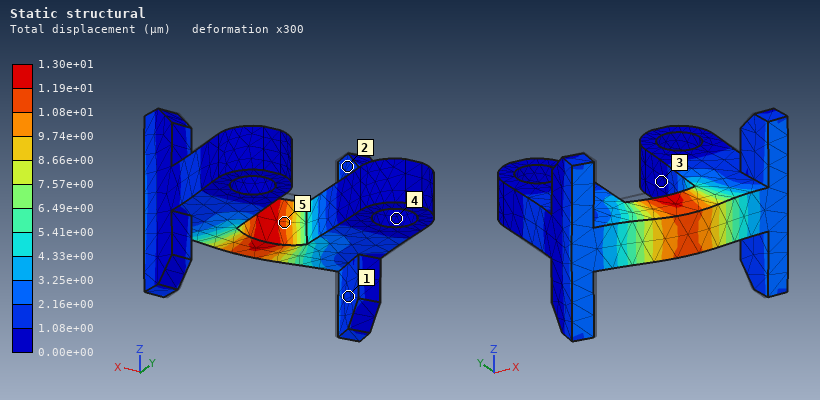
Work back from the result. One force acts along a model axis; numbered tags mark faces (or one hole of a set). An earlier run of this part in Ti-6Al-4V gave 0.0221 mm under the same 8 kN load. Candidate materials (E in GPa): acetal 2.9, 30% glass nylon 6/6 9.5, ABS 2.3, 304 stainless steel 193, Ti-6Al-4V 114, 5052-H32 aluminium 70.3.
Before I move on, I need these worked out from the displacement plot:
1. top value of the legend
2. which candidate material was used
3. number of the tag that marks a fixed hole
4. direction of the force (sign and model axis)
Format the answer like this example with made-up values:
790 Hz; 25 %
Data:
1.30e+01 µm; 304 stainless steel; 4; -Y
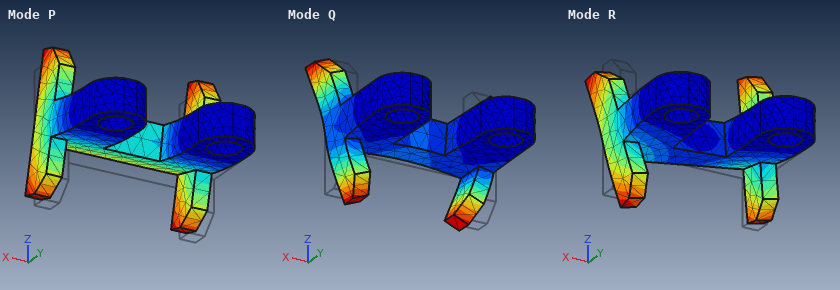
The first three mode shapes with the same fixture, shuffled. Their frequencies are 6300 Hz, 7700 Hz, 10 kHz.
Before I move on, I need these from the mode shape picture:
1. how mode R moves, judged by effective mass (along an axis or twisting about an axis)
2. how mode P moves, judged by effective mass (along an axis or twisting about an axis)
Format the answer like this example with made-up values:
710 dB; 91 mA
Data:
twisting about Y; along Z
